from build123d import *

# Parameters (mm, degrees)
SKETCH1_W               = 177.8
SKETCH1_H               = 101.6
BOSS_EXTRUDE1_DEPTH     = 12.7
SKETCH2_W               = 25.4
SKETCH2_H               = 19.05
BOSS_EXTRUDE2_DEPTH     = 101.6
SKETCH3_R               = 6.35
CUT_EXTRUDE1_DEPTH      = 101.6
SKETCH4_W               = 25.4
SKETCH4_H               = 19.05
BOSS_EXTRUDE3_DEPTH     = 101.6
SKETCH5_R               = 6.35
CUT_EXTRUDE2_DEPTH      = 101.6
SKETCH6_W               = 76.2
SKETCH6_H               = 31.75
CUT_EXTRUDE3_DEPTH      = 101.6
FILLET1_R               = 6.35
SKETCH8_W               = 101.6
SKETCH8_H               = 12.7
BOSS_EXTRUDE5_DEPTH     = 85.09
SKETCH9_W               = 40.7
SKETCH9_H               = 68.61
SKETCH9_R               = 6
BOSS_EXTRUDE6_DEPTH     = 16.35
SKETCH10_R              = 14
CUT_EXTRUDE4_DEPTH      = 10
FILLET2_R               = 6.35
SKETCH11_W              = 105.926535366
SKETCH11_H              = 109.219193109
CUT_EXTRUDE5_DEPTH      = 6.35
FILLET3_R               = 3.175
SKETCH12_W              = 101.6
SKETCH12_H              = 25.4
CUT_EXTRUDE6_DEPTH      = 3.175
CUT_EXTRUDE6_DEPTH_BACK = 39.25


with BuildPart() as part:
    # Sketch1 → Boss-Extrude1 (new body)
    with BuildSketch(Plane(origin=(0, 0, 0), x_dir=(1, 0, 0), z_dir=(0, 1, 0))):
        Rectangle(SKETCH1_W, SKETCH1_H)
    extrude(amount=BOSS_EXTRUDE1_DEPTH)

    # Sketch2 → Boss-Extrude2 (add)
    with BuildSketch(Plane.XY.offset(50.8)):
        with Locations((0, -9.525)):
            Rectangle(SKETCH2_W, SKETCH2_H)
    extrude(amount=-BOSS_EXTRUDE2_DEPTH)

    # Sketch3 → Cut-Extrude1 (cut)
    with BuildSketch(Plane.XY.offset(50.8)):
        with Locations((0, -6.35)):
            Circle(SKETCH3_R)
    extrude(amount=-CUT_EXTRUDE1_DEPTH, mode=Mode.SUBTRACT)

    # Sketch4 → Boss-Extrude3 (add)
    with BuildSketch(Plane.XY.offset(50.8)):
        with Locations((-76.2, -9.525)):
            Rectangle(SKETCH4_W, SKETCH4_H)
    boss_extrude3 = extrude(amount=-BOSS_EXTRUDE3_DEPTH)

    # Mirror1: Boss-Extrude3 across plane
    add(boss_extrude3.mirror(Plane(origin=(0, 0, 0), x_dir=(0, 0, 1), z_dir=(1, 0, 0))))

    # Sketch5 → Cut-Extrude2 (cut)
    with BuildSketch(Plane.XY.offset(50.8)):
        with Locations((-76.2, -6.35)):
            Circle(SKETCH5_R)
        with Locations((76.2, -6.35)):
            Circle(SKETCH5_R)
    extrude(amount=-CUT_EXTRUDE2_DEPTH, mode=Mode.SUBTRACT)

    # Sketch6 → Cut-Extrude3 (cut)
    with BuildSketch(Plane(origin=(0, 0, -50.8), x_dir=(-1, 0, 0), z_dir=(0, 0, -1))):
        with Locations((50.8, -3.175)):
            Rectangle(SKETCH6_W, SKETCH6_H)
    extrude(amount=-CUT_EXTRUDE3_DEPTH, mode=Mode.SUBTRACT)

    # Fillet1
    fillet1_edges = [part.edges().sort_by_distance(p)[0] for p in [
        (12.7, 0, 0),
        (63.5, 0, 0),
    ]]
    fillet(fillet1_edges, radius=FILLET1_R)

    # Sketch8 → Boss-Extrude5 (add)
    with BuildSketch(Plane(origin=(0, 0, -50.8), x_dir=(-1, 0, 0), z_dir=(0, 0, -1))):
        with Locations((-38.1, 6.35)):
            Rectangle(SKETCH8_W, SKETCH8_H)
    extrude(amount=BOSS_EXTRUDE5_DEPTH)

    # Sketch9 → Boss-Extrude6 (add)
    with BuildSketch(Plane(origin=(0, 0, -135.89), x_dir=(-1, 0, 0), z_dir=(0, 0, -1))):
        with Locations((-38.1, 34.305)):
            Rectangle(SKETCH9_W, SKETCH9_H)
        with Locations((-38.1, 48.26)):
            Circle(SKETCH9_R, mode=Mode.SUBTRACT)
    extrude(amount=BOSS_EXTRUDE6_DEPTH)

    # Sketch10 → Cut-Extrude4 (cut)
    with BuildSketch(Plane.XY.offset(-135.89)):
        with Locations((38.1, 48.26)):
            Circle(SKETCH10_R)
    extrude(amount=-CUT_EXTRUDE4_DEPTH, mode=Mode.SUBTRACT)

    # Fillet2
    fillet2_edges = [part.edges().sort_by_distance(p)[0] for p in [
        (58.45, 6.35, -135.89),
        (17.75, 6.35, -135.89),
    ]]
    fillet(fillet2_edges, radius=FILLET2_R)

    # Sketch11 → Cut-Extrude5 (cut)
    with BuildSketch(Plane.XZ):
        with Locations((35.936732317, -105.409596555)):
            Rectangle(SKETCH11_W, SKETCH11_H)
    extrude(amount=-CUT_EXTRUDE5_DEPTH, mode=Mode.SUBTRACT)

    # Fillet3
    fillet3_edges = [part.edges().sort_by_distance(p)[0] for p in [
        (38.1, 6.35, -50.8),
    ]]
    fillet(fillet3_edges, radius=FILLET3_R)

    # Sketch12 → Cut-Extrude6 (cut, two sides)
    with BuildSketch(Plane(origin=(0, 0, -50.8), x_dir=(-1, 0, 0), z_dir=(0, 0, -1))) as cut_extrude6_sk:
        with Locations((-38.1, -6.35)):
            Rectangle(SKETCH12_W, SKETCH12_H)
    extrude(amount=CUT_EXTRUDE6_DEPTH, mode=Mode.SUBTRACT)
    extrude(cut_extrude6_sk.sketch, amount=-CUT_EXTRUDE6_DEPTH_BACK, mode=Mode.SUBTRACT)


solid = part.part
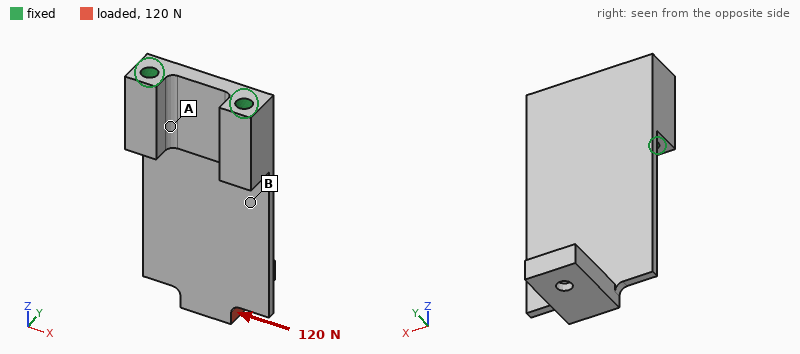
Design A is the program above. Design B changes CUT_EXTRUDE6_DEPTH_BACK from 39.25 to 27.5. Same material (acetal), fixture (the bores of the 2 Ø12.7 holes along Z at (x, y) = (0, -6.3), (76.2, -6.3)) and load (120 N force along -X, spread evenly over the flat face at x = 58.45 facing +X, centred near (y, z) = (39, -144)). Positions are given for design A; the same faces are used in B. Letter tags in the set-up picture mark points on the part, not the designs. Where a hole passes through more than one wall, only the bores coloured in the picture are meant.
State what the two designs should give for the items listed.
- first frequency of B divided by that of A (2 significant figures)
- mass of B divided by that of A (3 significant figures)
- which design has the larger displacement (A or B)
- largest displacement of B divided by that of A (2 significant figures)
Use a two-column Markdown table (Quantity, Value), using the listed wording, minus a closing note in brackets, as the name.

| Quantity | Value |
|---|---|
| first frequency of B divided by that of A | 1.2 |
| mass of B divided by that of A | 1.07 |
| which design has the larger displacement | A |
| largest displacement of B divided by that of A | 0.89 |
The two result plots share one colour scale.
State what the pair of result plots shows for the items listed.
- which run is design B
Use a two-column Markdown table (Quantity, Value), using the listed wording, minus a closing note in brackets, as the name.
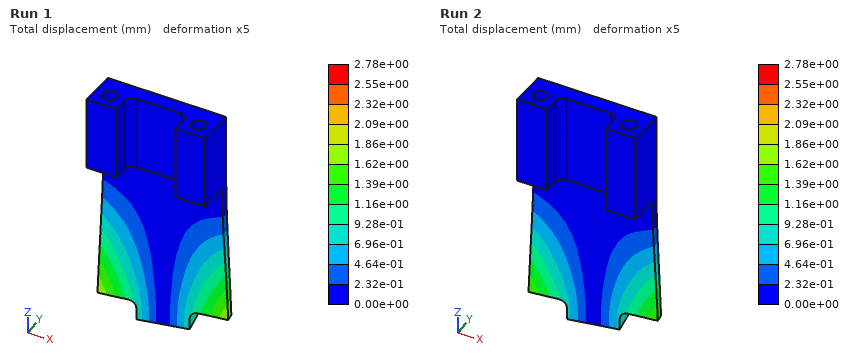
| Quantity | Value |
|---|---|
| which run is design B | Run 2 |
